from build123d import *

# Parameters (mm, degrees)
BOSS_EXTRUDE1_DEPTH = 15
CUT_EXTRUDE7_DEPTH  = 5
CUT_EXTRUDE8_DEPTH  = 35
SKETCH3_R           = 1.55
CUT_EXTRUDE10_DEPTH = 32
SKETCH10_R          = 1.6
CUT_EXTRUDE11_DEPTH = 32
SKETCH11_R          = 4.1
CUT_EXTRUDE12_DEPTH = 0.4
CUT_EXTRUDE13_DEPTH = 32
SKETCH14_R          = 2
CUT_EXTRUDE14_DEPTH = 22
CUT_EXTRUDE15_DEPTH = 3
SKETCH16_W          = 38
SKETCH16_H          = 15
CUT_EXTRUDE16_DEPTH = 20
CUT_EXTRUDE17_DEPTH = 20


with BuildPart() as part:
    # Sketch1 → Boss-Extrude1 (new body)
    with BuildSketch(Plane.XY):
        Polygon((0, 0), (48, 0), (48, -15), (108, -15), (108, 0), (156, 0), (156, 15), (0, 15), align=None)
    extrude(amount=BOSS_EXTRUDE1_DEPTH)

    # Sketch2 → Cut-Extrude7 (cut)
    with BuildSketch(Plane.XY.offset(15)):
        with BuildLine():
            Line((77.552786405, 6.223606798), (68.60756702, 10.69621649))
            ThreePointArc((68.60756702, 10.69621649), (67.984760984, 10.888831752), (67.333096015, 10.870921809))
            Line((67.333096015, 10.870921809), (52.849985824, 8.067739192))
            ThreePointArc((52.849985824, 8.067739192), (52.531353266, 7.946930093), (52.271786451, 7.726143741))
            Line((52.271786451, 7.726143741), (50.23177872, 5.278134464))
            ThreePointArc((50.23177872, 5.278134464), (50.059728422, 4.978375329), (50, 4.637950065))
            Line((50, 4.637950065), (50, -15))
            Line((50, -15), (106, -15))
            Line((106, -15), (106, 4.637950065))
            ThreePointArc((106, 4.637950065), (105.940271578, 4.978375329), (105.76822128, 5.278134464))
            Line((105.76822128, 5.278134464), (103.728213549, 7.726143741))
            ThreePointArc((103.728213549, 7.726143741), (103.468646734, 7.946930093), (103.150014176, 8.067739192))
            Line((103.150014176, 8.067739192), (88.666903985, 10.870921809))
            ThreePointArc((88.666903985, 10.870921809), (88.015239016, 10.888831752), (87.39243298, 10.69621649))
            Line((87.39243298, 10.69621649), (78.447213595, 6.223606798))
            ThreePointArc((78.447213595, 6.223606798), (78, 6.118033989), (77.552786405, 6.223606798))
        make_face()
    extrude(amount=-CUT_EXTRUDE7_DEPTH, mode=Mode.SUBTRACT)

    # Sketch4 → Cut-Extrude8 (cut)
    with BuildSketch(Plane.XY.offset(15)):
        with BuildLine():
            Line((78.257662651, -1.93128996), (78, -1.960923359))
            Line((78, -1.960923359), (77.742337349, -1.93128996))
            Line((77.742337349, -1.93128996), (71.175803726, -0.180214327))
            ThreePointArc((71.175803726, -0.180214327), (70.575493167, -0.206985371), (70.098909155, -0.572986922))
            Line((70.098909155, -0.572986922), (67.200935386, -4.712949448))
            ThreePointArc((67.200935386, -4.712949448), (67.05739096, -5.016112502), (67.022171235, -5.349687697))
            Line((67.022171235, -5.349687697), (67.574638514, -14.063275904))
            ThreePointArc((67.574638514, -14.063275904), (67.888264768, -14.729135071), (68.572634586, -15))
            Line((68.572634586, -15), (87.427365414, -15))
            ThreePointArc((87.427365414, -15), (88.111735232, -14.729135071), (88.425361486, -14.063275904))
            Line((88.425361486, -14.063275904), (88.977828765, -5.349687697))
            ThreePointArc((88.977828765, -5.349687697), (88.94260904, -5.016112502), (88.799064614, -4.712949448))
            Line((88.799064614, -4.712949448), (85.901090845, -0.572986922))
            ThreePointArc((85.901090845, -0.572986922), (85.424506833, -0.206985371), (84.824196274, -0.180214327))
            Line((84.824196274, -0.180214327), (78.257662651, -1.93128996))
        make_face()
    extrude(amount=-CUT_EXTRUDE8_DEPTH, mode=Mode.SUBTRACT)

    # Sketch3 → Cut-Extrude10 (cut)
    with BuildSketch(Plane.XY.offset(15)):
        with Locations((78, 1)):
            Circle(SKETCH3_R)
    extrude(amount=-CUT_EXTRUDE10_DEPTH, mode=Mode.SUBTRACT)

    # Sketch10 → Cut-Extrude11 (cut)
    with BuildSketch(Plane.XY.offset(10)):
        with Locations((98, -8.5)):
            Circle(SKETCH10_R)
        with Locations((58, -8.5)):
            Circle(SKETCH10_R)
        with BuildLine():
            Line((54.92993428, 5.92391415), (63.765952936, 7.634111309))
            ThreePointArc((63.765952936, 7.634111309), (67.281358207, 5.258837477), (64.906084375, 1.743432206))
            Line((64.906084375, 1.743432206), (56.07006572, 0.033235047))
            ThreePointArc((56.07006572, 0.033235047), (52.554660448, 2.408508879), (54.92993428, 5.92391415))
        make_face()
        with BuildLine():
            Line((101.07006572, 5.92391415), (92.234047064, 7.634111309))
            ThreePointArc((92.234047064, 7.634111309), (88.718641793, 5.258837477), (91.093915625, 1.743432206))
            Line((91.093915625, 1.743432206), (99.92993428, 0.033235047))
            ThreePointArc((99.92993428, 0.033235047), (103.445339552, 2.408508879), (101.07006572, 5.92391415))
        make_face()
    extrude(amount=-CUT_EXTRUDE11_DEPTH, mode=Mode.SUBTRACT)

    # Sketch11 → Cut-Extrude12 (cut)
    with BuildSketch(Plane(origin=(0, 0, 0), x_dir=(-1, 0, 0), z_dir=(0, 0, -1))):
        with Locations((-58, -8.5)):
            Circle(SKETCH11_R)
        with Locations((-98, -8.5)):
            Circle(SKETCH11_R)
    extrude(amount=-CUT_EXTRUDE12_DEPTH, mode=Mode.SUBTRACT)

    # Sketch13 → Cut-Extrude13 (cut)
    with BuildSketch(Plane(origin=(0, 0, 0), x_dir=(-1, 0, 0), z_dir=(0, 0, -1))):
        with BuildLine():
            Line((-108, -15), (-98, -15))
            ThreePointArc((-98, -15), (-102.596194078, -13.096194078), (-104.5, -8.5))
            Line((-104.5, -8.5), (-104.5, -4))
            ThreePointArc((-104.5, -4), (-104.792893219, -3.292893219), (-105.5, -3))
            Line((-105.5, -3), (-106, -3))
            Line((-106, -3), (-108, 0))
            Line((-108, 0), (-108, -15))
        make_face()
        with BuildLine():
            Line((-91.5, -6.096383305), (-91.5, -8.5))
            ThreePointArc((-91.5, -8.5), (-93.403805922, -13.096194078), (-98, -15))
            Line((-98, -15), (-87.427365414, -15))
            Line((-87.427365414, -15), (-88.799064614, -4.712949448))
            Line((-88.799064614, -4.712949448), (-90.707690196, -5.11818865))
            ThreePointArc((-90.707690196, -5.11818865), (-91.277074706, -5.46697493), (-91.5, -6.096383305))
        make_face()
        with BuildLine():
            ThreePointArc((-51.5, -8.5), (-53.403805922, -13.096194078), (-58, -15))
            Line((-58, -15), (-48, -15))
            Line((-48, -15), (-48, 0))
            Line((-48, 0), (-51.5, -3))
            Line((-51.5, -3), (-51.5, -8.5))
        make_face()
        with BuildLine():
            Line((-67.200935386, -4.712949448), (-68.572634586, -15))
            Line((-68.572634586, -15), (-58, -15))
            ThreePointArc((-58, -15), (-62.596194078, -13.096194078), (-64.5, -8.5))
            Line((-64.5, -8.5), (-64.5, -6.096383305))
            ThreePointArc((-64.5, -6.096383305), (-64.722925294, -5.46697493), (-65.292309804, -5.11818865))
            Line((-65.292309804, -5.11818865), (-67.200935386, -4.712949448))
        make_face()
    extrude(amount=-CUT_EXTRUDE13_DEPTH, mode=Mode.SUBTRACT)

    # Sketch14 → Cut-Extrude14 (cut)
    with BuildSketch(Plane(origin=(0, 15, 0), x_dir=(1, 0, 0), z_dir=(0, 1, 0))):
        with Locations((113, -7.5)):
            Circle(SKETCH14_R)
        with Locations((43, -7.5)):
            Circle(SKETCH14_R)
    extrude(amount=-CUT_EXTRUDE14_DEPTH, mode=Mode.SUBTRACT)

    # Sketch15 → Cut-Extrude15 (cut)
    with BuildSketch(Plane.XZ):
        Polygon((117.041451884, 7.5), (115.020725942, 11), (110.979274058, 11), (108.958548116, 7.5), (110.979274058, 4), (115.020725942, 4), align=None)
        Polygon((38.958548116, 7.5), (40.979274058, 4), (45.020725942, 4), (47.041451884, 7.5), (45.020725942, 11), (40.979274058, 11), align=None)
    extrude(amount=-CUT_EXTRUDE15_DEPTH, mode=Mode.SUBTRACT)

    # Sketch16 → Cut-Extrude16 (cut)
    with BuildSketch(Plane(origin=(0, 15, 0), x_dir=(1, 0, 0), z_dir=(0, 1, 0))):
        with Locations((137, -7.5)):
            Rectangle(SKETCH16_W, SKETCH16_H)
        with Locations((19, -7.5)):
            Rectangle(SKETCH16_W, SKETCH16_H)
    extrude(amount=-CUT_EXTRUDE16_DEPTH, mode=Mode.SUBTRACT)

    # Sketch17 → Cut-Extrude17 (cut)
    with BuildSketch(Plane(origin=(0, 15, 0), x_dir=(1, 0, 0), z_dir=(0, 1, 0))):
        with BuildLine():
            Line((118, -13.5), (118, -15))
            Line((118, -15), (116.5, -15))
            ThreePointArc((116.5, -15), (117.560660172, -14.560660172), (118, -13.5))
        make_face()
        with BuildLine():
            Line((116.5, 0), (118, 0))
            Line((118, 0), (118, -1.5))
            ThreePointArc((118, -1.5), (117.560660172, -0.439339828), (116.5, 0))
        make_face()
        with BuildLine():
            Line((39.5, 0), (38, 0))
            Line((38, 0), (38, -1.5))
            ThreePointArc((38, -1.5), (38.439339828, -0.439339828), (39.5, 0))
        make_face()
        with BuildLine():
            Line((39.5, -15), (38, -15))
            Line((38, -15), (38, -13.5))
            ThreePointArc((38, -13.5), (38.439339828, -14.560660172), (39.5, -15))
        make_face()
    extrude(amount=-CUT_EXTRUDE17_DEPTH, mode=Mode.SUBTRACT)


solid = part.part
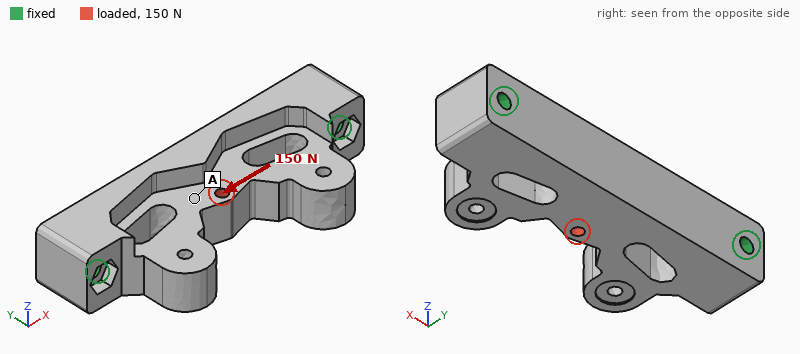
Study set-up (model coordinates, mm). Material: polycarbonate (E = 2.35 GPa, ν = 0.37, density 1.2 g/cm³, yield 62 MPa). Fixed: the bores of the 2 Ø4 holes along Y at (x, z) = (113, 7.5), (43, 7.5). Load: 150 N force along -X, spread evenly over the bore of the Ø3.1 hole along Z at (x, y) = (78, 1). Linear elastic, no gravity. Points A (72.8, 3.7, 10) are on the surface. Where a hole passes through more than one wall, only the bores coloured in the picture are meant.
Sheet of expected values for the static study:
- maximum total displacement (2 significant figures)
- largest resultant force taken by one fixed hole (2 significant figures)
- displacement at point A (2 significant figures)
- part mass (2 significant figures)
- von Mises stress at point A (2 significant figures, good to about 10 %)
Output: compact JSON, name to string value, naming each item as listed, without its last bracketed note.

{"maximum total displacement": "21 µm", "largest resultant force taken by one fixed hole": "78 N", "displacement at point A": "14 µm", "part mass": "21 g", "von Mises stress at point A": "0.60 MPa"}
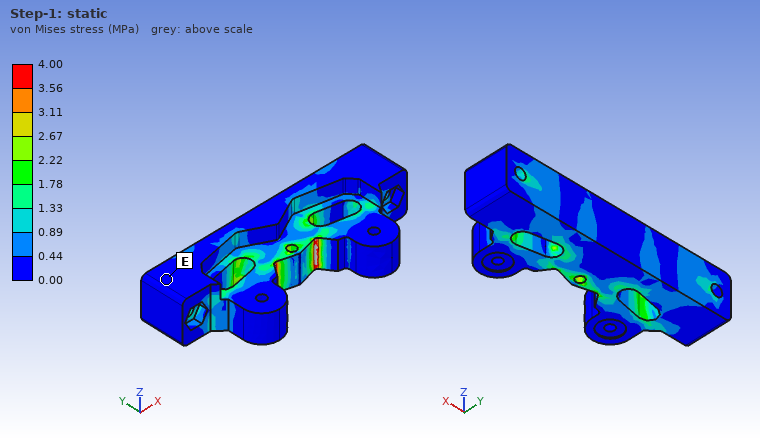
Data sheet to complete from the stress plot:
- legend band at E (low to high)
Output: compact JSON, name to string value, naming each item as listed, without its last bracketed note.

{"legend band at E": "0.00 to 0.44 MPa"}
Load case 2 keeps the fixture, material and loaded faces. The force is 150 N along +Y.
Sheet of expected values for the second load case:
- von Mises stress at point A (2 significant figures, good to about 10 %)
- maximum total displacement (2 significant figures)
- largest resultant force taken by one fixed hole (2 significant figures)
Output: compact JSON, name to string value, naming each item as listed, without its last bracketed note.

{"von Mises stress at point A": "1.5 MPa", "maximum total displacement": "91 µm", "largest resultant force taken by one fixed hole": "75 N"}
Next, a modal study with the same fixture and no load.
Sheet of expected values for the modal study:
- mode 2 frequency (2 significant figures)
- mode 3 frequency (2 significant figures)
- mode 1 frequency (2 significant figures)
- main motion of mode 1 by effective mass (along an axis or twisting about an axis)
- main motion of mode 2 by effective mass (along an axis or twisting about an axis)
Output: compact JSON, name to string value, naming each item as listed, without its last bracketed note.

{"mode 2 frequency": "2400 Hz", "mode 3 frequency": "3200 Hz", "mode 1 frequency": "2100 Hz", "main motion of mode 1 by effective mass": "along Z", "main motion of mode 2 by effective mass": "along Y"}
